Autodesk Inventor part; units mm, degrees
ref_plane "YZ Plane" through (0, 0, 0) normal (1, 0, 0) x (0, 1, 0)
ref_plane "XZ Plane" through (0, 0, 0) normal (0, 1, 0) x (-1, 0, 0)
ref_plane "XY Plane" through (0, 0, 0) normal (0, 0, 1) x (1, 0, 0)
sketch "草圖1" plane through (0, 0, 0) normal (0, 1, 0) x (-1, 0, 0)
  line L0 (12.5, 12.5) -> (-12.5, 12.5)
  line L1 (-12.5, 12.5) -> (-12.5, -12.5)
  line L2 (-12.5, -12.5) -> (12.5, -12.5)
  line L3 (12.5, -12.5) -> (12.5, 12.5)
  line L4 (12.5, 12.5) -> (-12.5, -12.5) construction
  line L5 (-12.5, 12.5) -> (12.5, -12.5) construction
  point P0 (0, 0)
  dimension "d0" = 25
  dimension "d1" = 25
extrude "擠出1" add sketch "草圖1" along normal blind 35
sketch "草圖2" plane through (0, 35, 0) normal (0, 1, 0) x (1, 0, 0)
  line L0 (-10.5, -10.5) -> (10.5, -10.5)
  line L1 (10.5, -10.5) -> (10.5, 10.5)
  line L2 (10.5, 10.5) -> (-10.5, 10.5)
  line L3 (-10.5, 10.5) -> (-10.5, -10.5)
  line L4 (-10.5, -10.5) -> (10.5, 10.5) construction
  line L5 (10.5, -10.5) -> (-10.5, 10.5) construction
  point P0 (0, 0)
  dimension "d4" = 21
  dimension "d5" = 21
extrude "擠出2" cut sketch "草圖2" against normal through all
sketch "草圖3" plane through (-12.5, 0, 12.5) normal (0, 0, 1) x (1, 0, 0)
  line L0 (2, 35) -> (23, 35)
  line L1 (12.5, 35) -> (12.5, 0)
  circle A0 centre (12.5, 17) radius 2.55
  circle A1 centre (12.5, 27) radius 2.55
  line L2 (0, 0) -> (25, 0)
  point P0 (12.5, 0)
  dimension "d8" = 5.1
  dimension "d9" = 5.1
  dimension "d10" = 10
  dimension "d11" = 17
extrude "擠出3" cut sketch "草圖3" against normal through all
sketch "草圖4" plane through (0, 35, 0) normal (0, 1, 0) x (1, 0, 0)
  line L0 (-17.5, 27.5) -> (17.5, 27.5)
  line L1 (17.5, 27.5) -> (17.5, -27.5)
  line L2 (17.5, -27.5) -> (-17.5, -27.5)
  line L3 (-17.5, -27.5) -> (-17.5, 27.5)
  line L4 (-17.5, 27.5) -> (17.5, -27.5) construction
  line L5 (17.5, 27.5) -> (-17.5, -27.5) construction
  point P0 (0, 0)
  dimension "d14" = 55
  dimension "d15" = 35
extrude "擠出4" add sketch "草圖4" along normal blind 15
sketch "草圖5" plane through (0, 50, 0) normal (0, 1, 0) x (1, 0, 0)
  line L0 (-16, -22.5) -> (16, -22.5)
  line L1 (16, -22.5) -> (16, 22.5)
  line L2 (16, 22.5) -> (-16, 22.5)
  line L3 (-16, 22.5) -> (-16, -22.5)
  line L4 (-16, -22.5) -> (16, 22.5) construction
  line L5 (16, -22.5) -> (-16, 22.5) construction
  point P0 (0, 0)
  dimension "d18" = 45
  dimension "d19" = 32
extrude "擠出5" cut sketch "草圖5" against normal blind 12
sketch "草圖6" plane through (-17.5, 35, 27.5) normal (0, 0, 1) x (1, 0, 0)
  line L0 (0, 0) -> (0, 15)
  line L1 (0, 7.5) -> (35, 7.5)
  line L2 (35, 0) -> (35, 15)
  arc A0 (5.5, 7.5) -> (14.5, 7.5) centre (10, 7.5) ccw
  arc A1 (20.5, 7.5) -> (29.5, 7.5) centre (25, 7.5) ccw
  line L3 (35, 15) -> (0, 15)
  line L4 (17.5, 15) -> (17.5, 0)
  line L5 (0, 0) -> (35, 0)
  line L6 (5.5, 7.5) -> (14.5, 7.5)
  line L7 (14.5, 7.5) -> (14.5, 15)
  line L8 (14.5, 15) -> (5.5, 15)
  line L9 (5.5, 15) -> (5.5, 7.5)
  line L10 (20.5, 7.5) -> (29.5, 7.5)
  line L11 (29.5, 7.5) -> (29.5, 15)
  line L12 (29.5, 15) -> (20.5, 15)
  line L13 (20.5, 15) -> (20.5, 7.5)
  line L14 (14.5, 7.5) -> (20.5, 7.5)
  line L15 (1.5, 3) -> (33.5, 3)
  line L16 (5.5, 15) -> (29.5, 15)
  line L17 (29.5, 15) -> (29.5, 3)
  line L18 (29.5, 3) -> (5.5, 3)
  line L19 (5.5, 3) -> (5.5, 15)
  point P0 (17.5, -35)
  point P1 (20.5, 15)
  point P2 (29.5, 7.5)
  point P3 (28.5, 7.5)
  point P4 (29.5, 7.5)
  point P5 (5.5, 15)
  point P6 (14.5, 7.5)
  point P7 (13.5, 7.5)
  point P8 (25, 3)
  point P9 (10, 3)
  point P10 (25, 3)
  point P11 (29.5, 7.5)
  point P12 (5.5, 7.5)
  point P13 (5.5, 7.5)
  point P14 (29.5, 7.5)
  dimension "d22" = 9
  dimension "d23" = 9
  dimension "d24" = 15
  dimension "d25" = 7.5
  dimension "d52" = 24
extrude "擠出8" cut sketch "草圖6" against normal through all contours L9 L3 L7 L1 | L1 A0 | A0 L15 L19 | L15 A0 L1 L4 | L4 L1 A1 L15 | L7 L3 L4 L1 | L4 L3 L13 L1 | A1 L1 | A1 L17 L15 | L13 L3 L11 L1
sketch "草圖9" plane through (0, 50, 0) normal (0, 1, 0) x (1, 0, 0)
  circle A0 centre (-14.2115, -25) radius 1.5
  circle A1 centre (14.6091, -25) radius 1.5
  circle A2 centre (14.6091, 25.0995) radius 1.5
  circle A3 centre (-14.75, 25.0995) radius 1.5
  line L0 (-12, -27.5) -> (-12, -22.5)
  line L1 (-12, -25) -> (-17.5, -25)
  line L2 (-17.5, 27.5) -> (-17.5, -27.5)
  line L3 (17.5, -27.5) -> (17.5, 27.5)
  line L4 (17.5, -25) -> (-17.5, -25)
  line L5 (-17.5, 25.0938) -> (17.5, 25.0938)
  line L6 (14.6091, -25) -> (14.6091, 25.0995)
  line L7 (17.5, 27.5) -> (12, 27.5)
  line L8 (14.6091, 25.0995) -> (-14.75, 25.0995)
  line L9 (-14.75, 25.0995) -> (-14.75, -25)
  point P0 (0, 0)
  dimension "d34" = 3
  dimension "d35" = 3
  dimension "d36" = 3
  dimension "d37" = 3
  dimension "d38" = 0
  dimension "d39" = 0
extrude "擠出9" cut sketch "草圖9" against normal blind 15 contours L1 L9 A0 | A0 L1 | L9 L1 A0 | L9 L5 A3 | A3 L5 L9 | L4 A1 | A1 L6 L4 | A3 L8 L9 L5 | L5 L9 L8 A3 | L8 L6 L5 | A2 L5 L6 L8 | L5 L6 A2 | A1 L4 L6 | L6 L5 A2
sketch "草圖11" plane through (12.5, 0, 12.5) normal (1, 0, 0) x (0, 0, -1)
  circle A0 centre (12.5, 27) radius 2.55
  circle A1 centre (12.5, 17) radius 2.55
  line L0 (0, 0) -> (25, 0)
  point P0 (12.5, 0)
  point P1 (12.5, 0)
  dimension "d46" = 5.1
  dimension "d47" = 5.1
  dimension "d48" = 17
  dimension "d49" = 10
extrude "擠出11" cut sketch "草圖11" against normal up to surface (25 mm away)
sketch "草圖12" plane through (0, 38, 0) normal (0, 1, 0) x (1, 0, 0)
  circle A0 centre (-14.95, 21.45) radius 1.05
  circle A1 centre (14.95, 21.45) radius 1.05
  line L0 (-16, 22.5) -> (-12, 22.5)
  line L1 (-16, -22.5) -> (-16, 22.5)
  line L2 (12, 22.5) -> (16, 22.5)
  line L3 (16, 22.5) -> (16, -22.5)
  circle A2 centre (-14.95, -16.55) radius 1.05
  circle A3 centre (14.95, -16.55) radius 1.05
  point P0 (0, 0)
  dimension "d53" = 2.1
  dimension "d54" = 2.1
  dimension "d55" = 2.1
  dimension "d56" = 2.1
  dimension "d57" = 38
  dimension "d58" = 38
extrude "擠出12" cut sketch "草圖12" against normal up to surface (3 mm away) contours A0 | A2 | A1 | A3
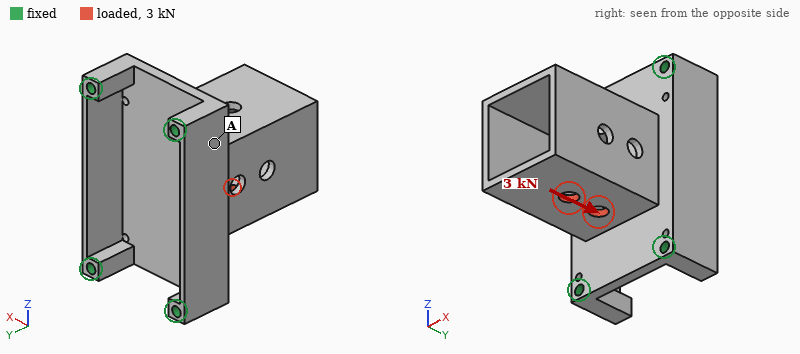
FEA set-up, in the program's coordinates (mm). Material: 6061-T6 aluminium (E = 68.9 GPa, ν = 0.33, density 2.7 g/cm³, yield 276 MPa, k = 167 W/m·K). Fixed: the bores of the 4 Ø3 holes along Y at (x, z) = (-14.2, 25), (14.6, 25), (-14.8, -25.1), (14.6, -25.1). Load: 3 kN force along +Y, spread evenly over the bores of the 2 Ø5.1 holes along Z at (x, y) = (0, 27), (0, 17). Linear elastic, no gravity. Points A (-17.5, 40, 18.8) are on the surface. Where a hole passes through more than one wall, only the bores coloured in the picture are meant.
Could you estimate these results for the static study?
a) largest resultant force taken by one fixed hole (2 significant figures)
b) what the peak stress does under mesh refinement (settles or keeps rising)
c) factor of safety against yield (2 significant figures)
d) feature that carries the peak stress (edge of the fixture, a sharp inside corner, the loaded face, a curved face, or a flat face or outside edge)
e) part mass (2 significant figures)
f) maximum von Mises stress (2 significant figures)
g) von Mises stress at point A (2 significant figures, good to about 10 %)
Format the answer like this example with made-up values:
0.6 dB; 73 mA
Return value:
1.2 kN; settles; 0.74; a curved face; 39 g; 370 MPa; 26 MPa
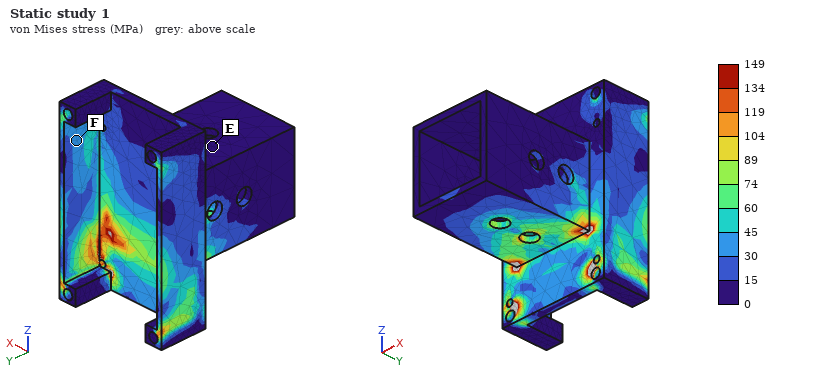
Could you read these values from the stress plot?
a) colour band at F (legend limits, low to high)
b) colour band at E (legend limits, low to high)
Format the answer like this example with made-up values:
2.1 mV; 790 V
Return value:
30 to 45 MPa; 0 to 15 MPa
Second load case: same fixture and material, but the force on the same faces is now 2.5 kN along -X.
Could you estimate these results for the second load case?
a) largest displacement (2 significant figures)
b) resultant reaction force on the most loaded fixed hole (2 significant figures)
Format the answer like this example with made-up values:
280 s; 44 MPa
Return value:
0.15 mm; 1.3 kN
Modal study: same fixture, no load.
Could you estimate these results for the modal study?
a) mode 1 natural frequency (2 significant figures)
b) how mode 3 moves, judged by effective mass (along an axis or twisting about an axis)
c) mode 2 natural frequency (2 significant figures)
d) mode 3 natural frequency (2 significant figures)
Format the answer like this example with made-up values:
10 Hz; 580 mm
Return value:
5600 Hz; along Y; 5700 Hz; 7600 Hz
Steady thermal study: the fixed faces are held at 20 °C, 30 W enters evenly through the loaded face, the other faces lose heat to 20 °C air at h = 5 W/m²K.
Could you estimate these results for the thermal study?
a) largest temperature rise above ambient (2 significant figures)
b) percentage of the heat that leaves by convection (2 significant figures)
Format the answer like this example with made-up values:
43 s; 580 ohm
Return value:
46 K; 3.4 %
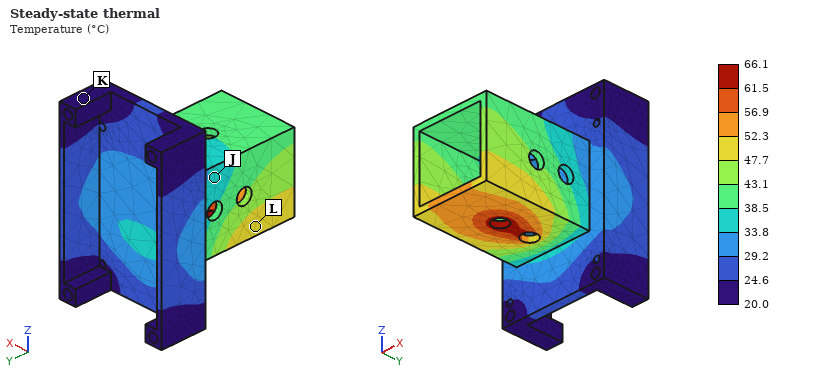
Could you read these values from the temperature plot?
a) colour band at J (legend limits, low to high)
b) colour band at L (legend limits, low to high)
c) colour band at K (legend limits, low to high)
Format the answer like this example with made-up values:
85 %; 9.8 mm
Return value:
33.8 to 38.5 °C; 47.7 to 52.3 °C; 20.0 to 24.6 °C
